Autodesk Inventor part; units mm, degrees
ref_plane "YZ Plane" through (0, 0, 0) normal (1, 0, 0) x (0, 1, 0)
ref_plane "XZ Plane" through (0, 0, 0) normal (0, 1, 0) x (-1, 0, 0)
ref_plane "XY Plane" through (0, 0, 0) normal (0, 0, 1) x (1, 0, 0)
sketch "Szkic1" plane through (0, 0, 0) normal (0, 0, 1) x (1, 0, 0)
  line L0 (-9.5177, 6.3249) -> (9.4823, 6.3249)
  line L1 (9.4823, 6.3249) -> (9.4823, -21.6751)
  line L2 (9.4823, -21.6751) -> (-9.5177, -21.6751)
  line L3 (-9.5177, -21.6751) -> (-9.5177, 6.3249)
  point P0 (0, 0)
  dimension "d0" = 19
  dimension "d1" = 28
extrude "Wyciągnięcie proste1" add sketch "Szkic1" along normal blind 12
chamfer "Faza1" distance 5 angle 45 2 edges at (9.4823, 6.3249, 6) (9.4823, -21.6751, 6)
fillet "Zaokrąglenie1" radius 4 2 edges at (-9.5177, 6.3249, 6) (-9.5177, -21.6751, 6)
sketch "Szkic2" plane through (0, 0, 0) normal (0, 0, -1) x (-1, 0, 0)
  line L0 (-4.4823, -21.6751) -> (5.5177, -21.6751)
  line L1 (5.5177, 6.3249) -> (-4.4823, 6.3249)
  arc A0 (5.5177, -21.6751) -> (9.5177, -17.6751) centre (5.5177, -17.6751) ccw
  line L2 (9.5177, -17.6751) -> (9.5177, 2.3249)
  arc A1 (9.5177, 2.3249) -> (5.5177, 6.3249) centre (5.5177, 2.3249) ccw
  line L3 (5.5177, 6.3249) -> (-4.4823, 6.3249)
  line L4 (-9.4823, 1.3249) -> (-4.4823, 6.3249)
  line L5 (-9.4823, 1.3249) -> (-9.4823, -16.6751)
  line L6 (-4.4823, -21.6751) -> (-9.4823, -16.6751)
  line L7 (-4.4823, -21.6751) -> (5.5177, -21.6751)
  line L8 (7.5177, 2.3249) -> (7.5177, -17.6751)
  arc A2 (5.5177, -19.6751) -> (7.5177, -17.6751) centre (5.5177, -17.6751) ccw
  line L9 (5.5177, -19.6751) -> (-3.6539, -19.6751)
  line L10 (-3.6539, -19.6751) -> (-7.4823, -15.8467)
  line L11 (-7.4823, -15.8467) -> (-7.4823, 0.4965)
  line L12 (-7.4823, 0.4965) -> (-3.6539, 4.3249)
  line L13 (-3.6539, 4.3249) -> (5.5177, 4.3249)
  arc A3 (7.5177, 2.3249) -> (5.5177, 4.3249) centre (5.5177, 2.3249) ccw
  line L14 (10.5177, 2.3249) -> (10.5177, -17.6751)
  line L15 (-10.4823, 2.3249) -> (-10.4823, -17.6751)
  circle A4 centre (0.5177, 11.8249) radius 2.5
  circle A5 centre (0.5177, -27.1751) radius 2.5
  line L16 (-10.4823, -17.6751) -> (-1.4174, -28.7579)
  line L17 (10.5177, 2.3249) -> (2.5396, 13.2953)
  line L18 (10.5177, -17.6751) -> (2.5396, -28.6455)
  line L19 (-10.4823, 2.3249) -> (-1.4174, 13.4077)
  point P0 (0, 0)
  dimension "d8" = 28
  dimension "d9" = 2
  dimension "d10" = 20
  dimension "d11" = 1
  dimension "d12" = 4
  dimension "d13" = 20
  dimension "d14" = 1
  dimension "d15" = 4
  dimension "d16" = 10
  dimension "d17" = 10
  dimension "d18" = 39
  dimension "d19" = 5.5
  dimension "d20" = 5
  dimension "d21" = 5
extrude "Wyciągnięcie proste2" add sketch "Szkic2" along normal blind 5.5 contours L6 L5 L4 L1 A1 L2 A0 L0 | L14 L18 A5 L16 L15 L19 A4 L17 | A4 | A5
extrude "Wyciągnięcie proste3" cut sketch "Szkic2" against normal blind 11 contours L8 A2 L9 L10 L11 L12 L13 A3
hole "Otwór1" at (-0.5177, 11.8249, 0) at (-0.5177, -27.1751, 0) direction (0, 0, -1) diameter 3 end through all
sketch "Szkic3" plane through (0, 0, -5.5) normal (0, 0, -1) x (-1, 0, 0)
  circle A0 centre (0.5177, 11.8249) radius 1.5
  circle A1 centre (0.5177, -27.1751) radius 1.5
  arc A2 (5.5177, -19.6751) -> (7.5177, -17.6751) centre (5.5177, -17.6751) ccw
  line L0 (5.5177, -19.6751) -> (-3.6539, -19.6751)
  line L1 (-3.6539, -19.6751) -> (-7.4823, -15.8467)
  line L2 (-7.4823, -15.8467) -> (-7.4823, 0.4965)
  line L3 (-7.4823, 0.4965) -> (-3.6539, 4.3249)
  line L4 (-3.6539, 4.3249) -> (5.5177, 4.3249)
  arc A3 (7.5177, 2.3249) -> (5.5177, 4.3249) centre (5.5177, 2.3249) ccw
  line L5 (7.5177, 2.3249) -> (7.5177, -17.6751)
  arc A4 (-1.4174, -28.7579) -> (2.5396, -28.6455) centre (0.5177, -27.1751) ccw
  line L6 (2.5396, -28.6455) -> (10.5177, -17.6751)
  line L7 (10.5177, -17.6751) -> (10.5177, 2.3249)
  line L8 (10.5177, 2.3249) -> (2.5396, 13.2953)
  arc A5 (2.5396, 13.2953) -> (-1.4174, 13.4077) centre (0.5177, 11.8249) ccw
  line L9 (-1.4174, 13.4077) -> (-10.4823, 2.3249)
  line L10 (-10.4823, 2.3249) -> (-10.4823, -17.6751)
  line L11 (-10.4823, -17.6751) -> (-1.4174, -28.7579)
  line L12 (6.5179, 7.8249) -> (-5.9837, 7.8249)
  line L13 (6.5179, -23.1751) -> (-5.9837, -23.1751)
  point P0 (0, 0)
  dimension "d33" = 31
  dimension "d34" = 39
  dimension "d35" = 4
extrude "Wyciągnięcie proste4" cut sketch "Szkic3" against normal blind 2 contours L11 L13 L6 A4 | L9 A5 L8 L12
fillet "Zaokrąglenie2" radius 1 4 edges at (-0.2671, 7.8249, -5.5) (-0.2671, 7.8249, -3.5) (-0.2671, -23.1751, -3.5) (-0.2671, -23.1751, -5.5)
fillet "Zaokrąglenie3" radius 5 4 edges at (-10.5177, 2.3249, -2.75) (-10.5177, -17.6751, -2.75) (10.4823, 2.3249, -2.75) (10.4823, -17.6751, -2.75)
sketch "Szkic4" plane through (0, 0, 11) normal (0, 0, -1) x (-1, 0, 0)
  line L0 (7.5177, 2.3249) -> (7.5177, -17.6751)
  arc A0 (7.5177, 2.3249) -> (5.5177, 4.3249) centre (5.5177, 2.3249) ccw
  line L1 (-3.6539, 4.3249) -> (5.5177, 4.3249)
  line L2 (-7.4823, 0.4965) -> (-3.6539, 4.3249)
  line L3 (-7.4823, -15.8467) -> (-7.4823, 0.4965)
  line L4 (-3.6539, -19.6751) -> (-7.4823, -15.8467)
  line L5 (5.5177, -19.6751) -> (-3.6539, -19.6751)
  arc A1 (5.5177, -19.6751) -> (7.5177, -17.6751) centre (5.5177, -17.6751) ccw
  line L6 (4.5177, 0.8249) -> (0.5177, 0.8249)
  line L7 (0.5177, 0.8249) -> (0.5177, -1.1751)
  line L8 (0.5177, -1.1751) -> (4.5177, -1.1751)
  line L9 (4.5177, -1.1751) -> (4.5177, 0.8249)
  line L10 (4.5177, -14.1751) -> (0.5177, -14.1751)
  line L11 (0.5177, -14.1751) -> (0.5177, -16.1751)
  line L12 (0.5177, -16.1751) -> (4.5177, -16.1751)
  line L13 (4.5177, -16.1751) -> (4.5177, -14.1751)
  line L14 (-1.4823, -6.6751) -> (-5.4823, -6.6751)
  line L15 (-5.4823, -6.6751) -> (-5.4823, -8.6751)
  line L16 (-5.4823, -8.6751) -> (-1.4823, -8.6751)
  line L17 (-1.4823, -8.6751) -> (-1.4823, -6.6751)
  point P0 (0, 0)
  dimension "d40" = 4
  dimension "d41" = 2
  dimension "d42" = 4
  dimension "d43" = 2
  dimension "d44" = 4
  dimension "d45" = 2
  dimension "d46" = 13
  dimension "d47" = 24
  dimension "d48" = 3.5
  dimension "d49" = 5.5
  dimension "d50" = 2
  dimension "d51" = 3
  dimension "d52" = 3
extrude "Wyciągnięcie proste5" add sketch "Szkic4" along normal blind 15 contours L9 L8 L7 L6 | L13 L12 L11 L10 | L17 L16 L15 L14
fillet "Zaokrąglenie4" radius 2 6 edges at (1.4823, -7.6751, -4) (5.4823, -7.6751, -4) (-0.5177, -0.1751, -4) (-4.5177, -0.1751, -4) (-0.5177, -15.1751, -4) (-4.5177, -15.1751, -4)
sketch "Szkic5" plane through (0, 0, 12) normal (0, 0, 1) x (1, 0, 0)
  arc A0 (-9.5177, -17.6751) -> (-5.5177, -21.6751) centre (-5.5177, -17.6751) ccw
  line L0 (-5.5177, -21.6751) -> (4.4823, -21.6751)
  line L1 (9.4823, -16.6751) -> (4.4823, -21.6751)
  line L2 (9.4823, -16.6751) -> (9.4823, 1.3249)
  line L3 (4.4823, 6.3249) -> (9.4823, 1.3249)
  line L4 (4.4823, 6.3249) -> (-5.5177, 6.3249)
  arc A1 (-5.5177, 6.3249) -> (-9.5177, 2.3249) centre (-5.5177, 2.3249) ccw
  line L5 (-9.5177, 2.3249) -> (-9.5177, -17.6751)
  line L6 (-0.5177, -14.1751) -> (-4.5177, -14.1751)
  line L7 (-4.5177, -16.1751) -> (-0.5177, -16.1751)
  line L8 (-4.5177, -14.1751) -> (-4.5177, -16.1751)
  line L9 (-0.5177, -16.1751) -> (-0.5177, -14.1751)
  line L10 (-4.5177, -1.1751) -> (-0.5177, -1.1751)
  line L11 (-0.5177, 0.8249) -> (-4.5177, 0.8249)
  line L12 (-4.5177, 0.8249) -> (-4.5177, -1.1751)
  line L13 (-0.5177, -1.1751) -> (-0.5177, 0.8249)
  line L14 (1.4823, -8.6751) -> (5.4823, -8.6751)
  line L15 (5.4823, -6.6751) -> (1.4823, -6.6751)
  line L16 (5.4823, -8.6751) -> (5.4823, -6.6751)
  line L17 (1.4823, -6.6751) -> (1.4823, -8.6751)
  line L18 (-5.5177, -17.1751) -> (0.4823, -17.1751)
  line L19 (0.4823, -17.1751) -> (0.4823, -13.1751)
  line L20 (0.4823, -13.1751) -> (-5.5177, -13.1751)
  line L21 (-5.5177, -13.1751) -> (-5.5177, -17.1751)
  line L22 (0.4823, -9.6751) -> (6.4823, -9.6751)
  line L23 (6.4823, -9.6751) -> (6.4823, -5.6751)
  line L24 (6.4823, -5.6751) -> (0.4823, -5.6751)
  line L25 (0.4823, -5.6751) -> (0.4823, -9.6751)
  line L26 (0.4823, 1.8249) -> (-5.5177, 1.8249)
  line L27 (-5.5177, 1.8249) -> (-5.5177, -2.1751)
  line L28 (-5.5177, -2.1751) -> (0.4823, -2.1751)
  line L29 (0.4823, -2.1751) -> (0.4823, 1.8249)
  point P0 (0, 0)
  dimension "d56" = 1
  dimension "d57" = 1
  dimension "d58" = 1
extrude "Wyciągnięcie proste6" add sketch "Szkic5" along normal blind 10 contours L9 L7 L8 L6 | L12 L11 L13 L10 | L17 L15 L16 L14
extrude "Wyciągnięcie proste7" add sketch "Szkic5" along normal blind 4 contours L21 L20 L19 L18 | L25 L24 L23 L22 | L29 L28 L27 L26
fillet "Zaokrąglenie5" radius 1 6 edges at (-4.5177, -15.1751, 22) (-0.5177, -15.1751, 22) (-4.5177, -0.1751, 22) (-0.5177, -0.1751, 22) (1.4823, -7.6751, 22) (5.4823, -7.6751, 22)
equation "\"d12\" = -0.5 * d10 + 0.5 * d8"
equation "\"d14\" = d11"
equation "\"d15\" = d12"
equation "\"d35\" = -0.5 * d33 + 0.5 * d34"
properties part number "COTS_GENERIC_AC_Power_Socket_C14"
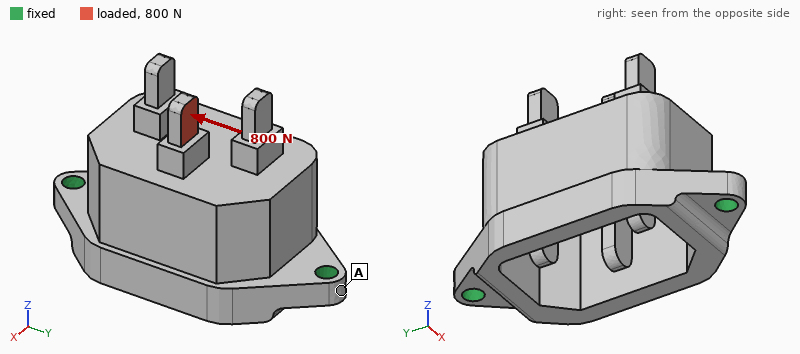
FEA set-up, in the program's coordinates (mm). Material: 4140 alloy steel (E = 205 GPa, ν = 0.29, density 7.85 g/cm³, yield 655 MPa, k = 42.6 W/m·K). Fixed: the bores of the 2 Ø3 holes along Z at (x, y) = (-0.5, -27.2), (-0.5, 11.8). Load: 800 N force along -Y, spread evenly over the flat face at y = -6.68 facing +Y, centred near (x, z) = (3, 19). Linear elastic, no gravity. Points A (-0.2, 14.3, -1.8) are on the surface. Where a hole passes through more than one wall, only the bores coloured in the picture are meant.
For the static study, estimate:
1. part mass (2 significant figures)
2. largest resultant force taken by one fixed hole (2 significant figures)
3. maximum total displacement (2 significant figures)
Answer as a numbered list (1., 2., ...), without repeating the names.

1. 37 g
2. 660 N
3. 0.18 mm
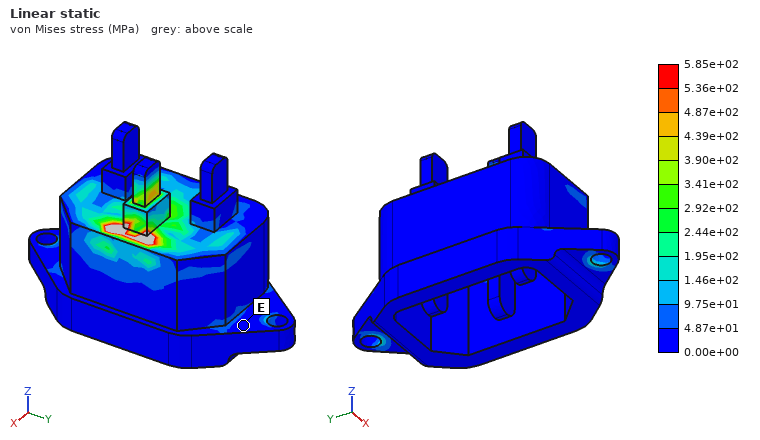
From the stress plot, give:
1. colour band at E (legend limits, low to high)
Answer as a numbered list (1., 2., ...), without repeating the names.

1. 0.00e+00 to 4.87e+01 MPa
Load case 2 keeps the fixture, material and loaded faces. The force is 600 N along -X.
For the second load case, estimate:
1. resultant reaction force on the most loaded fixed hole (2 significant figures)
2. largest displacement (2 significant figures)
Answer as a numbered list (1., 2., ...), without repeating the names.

1. 320 N
2. 0.17 mm
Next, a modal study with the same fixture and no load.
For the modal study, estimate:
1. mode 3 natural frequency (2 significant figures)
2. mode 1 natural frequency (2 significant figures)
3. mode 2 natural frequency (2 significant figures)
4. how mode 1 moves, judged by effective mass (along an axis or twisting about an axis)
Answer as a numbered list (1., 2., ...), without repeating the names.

1. 6300 Hz
2. 4800 Hz
3. 6100 Hz
4. along X
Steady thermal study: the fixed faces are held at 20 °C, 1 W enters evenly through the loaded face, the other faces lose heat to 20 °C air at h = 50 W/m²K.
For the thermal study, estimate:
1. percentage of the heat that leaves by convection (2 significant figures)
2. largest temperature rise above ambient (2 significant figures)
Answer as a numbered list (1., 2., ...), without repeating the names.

1. 55 %
2. 20 K
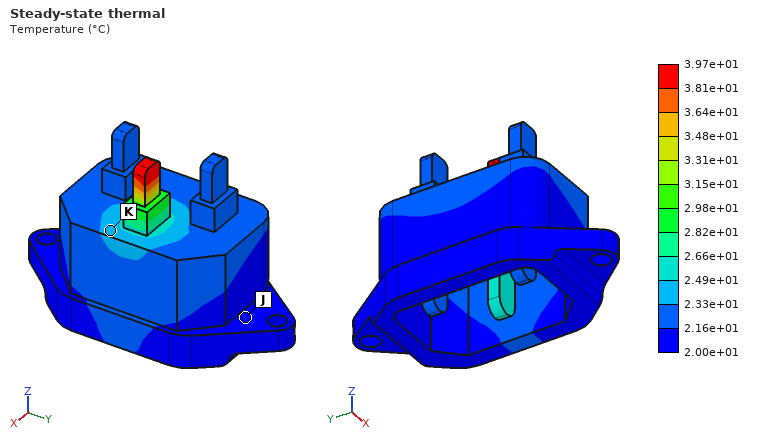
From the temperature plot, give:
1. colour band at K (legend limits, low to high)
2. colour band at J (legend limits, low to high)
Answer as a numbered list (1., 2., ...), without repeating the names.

1. 2.33e+01 to 2.49e+01 °C
2. 2.00e+01 to 2.16e+01 °C
